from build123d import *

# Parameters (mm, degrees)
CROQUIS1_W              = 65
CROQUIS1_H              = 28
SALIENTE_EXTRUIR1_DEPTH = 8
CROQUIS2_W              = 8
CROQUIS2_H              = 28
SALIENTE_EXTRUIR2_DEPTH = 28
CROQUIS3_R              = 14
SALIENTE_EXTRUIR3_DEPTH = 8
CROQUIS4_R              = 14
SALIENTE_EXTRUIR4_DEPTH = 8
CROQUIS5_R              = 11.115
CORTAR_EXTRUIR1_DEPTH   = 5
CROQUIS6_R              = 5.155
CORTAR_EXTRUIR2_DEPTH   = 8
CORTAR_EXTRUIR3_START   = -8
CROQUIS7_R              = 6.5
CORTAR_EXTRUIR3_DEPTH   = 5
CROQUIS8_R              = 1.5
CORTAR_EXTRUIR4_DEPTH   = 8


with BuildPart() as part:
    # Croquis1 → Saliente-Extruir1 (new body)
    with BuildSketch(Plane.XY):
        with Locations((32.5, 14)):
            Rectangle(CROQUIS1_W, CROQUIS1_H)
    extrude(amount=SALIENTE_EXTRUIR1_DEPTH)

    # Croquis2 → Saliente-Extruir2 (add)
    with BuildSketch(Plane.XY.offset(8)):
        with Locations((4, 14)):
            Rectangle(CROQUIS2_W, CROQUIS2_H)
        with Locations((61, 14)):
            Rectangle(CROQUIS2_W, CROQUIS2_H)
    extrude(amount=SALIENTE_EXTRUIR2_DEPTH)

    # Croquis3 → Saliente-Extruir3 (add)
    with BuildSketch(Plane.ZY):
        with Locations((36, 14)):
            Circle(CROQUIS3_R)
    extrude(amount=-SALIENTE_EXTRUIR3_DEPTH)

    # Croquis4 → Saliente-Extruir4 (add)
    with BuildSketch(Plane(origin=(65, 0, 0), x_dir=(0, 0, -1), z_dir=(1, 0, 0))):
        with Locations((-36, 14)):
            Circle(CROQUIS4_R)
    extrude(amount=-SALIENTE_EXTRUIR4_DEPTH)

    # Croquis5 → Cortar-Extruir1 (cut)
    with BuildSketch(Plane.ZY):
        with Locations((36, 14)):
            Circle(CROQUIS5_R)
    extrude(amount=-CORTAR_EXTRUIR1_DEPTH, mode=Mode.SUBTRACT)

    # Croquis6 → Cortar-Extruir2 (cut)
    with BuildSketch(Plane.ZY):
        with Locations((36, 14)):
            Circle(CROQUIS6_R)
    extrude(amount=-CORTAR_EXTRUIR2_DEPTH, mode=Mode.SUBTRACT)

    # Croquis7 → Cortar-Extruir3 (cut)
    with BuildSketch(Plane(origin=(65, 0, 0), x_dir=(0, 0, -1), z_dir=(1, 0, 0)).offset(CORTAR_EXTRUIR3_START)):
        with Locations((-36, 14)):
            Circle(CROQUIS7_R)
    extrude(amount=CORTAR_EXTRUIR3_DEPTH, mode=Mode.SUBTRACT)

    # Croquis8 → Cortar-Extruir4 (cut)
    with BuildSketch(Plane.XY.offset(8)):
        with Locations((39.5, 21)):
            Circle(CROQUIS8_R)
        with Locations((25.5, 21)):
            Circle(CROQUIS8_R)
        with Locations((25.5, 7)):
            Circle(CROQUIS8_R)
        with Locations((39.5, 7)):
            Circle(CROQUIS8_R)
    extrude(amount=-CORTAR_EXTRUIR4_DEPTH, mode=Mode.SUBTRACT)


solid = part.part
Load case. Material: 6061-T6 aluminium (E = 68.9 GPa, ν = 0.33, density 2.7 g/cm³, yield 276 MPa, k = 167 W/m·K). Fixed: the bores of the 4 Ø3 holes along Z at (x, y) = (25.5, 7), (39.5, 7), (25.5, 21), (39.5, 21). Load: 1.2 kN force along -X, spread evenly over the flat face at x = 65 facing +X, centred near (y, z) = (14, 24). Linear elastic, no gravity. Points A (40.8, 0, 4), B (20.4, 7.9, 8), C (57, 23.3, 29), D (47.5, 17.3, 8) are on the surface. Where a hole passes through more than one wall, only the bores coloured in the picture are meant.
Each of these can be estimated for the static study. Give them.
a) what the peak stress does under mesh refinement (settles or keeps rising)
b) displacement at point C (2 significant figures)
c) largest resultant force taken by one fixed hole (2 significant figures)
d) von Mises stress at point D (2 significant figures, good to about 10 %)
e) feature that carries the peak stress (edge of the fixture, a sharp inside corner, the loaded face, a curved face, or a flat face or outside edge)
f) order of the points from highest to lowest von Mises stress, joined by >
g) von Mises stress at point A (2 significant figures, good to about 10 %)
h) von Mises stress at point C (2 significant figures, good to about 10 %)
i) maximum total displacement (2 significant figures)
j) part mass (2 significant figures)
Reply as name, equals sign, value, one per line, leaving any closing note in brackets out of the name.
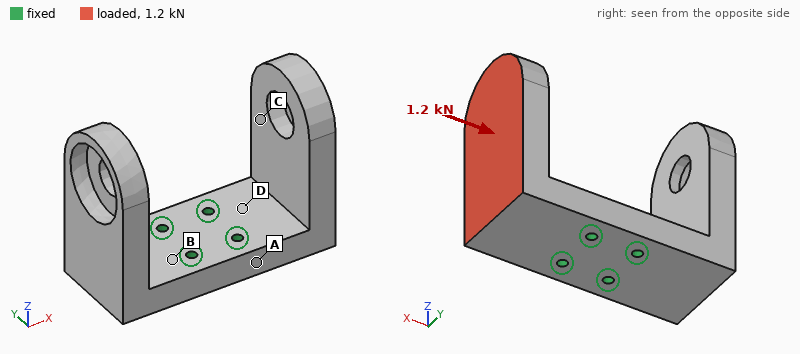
what the peak stress does under mesh refinement = keeps rising
displacement at point C = 0.20 mm
largest resultant force taken by one fixed hole = 570 N
von Mises stress at point D = 79 MPa
feature that carries the peak stress = edge of the fixture
order of the points from highest to lowest von Mises stress, joined by > = D > A > C > B
von Mises stress at point A = 28 MPa
von Mises stress at point C = 19 MPa
maximum total displacement = 0.41 mm
part mass = 78 g
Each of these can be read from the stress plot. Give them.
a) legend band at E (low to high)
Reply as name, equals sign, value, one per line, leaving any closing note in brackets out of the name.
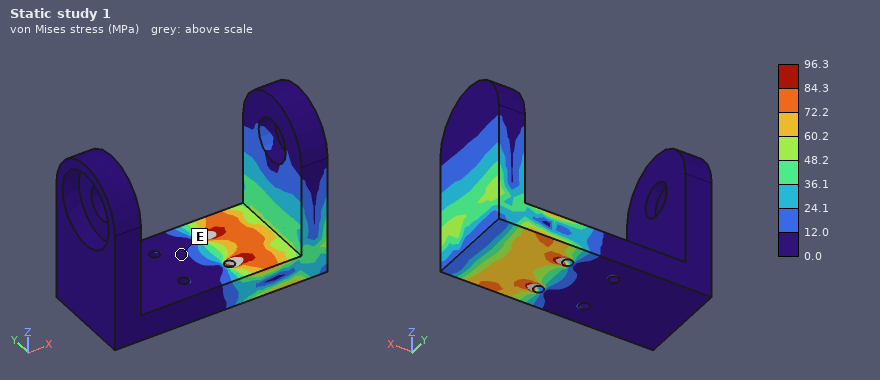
legend band at E = 0.0 to 12.0 MPa
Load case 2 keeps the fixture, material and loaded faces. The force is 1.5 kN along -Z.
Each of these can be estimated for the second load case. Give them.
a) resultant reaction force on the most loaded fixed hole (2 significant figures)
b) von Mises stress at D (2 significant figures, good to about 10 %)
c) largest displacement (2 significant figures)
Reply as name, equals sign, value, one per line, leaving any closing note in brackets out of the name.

resultant reaction force on the most loaded fixed hole = 1.1 kN
von Mises stress at D = 80 MPa
largest displacement = 0.33 mm
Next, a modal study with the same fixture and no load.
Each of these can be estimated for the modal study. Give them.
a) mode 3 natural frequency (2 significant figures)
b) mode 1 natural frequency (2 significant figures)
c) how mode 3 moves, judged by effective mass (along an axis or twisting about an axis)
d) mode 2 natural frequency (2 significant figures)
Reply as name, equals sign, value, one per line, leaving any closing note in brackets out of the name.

mode 3 natural frequency = 3200 Hz
mode 1 natural frequency = 2100 Hz
how mode 3 moves, judged by effective mass = along Y
mode 2 natural frequency = 2400 Hz
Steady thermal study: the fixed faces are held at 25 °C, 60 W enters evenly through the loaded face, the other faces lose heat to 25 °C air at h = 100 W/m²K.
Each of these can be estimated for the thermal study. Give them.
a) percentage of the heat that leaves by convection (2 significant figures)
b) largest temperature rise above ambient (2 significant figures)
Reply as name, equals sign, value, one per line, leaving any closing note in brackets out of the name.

percentage of the heat that leaves by convection = 20 %
largest temperature rise above ambient = 52 K
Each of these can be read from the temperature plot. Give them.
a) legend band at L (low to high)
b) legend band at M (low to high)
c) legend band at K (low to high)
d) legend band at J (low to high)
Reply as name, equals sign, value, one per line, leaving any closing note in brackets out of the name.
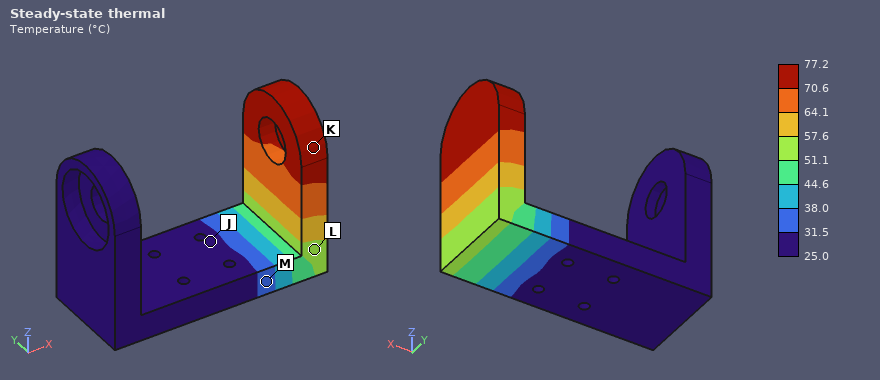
legend band at L = 51.1 to 57.6 °C
legend band at M = 31.5 to 38.0 °C
legend band at K = 70.6 to 77.2 °C
legend band at J = 25.0 to 31.5 °C
